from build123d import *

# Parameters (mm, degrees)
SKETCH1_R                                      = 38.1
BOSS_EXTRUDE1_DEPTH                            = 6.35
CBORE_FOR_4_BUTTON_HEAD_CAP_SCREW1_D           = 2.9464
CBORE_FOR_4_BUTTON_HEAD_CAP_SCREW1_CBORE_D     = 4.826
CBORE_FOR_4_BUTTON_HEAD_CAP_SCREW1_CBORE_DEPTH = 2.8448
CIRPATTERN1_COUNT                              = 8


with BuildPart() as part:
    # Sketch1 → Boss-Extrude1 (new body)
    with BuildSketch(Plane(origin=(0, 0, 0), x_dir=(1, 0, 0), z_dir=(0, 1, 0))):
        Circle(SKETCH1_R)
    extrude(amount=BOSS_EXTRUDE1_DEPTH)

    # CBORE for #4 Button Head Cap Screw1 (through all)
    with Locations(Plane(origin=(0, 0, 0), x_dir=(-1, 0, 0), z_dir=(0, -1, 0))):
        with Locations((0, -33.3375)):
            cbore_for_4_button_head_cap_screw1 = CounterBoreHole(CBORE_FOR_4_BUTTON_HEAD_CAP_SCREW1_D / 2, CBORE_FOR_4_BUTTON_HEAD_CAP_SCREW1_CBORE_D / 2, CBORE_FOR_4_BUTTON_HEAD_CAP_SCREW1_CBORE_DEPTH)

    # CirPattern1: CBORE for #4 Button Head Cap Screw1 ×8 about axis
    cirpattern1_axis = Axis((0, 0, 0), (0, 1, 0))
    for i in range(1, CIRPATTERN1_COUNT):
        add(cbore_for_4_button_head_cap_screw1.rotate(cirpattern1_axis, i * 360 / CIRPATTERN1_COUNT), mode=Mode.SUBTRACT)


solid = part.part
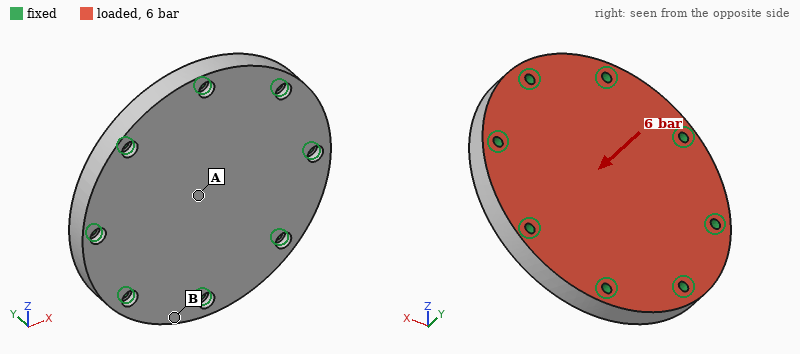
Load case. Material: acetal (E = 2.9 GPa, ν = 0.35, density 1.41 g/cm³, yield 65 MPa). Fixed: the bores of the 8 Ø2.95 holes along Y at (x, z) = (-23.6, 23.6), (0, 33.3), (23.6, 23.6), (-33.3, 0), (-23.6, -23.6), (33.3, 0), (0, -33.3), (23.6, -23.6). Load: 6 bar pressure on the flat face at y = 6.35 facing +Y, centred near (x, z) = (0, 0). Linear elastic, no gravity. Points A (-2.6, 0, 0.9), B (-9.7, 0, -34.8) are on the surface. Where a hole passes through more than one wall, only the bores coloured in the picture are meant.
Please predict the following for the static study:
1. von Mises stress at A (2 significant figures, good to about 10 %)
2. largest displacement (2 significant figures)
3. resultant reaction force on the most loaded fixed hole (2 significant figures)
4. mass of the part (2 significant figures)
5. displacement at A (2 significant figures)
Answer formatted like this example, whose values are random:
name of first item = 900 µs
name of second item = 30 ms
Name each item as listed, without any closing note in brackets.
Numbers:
von Mises stress at A = 13 MPa
largest displacement = 0.36 mm
resultant reaction force on the most loaded fixed hole = 380 N
mass of the part = 40 g
displacement at A = 0.35 mm
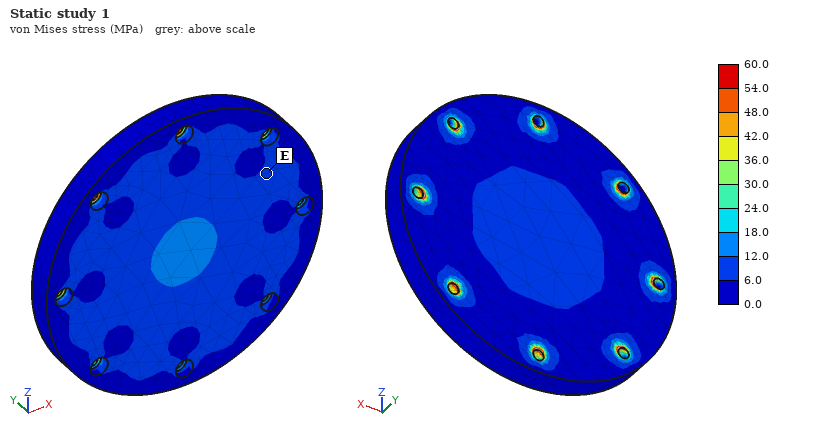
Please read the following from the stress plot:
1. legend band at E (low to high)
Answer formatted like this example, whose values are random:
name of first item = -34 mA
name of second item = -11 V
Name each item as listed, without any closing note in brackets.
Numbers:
legend band at E = 6.0 to 12.0 MPa
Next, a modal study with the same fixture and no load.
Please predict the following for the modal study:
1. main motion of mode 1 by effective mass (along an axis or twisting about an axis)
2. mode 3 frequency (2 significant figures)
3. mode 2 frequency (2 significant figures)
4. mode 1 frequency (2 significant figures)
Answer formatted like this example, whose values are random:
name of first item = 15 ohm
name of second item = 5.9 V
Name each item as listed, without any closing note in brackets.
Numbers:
main motion of mode 1 by effective mass = along Y
mode 3 frequency = 5500 Hz
mode 2 frequency = 5500 Hz
mode 1 frequency = 2600 Hz
